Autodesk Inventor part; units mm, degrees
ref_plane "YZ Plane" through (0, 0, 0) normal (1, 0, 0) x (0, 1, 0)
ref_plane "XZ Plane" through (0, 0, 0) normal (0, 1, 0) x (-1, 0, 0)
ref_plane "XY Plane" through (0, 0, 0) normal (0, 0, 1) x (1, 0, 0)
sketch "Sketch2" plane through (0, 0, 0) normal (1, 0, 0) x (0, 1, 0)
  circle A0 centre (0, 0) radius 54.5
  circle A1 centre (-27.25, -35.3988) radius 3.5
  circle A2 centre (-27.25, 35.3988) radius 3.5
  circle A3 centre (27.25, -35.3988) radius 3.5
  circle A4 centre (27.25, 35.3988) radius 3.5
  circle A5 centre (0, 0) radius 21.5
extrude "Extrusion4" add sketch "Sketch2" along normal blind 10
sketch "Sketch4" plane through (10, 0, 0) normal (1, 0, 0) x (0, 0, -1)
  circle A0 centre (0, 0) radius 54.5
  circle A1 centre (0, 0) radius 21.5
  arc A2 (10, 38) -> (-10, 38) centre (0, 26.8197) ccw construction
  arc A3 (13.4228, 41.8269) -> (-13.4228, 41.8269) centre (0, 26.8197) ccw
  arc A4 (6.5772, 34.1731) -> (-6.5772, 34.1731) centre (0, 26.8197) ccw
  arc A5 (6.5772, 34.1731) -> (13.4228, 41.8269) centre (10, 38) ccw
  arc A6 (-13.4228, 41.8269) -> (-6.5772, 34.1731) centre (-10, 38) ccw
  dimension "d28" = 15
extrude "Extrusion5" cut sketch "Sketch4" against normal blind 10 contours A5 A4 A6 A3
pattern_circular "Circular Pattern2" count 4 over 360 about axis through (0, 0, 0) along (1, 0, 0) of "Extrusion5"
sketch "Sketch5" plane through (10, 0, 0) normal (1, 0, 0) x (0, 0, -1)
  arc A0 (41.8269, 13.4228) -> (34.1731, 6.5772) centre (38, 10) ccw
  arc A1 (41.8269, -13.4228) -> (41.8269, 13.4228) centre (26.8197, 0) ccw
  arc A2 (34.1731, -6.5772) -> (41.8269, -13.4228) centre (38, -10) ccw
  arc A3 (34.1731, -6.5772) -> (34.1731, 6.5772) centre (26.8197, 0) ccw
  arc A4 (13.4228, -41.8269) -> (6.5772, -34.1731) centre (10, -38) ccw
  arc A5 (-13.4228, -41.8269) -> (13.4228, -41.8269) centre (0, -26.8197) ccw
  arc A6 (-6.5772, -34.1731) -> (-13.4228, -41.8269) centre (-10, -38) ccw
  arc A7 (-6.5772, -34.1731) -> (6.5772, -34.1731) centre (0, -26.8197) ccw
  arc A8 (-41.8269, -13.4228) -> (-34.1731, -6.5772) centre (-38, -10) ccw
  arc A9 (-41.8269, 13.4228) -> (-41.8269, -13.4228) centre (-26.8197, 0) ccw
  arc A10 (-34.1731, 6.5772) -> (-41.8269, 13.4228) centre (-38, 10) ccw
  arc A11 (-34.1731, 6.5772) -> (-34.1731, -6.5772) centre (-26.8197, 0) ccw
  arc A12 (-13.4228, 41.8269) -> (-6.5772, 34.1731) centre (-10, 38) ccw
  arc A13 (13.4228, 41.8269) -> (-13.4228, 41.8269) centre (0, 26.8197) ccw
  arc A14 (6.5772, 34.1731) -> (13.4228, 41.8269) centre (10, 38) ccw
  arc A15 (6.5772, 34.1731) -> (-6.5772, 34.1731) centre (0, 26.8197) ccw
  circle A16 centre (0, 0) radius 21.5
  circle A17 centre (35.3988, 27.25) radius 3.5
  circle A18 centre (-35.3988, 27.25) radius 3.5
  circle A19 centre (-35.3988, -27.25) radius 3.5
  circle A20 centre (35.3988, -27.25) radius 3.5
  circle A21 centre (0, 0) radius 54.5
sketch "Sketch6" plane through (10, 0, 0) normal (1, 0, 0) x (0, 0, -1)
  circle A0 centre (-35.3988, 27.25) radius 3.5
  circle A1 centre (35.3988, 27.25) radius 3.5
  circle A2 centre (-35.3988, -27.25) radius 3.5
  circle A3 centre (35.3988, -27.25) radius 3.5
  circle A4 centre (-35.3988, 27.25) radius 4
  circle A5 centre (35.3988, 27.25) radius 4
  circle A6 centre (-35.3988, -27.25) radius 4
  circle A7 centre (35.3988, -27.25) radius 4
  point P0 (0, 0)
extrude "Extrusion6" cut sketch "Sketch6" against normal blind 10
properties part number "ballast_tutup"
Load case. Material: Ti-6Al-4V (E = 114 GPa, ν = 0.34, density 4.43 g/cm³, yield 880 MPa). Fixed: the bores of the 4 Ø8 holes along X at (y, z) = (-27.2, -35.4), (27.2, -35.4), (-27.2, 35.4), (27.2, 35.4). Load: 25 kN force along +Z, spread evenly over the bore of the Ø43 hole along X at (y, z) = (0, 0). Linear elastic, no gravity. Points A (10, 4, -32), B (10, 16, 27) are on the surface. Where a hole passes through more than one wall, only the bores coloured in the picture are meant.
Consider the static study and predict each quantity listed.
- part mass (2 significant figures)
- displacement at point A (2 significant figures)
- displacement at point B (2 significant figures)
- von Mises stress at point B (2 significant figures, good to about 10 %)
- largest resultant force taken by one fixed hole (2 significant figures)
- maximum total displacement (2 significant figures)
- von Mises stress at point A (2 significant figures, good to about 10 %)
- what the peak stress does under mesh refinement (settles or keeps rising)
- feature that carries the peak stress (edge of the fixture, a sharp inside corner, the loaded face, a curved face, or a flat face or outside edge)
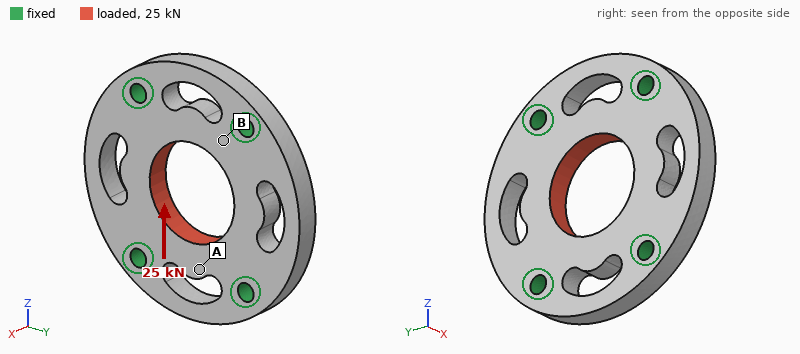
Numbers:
290 g
12 µm
5.3 µm
30 MPa
6.5 kN
13 µm
12 MPa
keeps rising
edge of the fixture
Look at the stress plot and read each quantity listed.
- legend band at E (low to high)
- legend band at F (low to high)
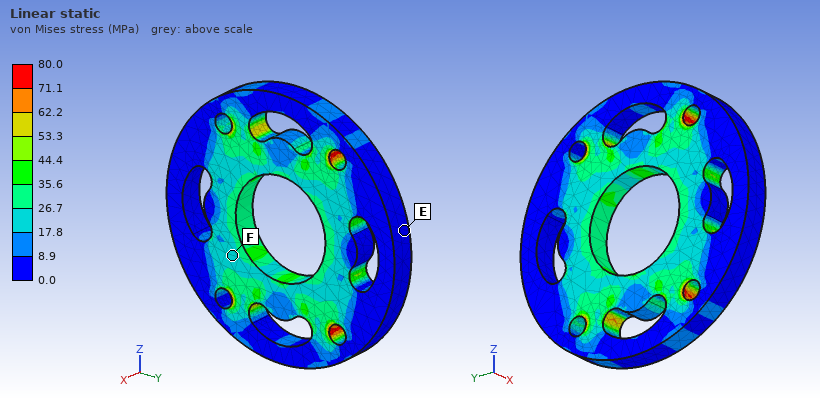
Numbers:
0.0 to 8.9 MPa
17.8 to 26.7 MPa
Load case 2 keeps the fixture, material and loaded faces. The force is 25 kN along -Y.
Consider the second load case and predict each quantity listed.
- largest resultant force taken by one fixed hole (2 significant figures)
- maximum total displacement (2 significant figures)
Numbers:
6.3 kN
20 µm
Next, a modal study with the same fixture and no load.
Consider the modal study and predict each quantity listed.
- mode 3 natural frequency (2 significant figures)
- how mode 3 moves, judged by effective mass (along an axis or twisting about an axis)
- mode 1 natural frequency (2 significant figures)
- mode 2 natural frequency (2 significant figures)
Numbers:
11 kHz
along X
7700 Hz
7800 Hz
